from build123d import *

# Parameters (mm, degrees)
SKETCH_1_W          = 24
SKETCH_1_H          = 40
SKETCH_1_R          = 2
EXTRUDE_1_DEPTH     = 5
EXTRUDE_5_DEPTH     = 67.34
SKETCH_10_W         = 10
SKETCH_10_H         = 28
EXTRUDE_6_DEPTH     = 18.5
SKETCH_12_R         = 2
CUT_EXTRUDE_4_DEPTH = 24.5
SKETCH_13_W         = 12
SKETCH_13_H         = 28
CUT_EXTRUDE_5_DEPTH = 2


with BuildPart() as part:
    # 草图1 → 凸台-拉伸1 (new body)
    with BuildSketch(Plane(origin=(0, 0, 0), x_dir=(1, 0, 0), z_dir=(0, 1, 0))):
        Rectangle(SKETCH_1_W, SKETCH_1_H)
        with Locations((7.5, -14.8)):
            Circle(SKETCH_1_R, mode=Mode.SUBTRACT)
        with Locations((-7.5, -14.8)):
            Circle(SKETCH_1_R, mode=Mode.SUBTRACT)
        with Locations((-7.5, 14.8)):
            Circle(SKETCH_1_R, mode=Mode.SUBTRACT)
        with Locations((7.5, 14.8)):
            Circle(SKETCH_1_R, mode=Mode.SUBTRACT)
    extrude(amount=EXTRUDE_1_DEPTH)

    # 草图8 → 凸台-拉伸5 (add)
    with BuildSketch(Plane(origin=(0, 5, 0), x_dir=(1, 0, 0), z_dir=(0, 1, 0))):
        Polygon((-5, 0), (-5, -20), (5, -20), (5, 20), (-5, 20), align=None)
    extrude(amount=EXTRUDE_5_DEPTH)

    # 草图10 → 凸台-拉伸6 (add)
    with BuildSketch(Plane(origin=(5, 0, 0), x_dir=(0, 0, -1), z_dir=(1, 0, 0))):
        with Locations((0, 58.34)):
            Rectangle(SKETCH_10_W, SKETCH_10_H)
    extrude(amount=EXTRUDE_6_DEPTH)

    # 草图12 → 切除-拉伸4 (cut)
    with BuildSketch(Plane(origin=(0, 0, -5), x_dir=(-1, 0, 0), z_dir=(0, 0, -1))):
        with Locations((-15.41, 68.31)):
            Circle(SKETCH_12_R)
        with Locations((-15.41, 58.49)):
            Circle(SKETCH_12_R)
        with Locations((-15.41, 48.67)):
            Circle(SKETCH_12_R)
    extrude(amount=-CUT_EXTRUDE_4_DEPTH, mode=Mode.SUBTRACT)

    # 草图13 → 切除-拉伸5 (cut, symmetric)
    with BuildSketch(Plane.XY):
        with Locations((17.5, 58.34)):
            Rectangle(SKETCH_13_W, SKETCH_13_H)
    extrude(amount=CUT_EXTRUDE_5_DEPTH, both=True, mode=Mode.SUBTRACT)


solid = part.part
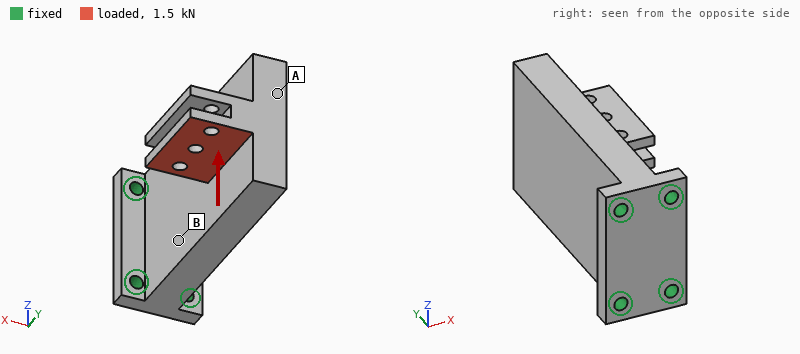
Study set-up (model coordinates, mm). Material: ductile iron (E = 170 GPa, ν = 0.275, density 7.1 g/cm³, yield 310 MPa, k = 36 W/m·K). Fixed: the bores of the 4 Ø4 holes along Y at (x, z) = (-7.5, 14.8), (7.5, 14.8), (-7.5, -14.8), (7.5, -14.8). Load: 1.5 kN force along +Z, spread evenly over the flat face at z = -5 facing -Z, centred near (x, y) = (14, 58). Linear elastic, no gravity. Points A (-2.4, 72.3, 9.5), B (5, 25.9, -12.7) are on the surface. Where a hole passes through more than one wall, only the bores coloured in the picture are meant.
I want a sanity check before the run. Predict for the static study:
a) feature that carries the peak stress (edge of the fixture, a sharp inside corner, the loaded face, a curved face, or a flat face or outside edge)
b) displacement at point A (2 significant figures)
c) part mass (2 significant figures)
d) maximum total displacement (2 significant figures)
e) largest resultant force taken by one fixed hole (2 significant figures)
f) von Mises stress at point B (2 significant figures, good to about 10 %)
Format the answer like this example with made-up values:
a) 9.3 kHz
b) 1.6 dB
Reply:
a) edge of the fixture
b) 24 µm
c) 250 g
d) 98 µm
e) 2.0 kN
f) 33 MPa
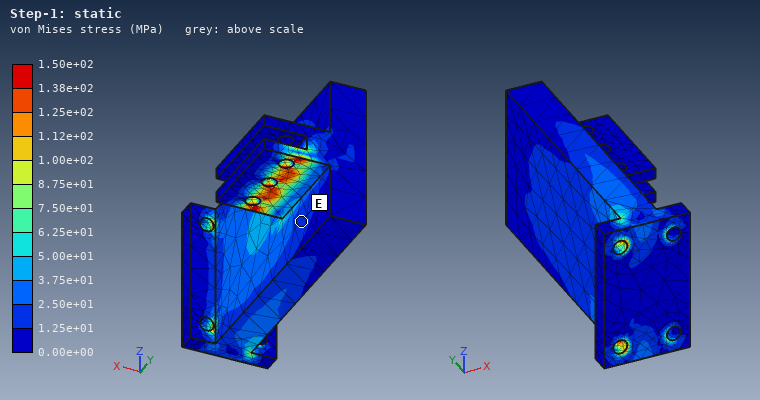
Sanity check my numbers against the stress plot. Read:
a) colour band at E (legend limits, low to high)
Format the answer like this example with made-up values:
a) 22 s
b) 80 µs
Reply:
a) 1.25e+01 to 2.50e+01 MPa
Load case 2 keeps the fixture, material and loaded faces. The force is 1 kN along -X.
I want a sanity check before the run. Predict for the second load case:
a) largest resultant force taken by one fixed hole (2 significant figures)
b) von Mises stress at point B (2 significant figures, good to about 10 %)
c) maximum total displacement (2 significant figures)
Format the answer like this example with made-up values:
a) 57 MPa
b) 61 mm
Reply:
a) 2.3 kN
b) 50 MPa
c) 0.18 mm
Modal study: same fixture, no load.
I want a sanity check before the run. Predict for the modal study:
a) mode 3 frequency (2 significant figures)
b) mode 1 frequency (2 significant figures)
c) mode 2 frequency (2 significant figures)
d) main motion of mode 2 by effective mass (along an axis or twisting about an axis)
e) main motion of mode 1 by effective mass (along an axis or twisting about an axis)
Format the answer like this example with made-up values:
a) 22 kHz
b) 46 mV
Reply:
a) 5000 Hz
b) 1300 Hz
c) 3800 Hz
d) along Z
e) along X
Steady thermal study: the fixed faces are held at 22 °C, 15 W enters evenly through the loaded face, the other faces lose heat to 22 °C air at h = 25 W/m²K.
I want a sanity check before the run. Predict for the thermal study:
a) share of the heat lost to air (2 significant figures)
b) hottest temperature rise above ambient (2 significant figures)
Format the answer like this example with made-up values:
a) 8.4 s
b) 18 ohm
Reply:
a) 44 %
b) 77 K
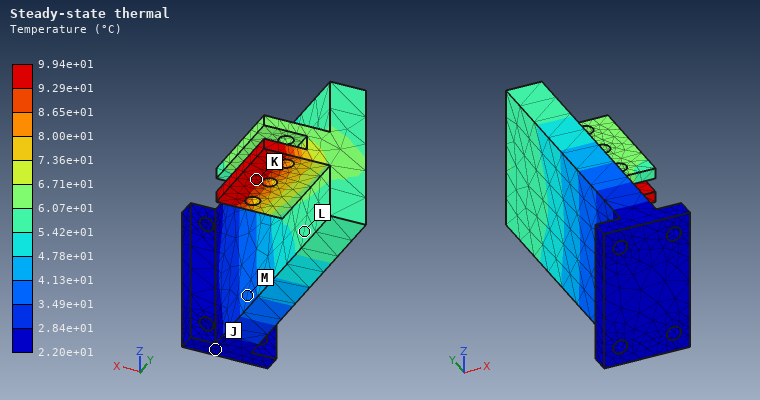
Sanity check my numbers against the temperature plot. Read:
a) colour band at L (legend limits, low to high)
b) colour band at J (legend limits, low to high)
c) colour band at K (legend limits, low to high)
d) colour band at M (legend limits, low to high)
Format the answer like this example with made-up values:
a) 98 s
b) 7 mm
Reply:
a) 5.42e+01 to 6.07e+01 °C
b) 2.20e+01 to 2.84e+01 °C
c) 9.29e+01 to 9.94e+01 °C
d) 3.49e+01 to 4.13e+01 °C
